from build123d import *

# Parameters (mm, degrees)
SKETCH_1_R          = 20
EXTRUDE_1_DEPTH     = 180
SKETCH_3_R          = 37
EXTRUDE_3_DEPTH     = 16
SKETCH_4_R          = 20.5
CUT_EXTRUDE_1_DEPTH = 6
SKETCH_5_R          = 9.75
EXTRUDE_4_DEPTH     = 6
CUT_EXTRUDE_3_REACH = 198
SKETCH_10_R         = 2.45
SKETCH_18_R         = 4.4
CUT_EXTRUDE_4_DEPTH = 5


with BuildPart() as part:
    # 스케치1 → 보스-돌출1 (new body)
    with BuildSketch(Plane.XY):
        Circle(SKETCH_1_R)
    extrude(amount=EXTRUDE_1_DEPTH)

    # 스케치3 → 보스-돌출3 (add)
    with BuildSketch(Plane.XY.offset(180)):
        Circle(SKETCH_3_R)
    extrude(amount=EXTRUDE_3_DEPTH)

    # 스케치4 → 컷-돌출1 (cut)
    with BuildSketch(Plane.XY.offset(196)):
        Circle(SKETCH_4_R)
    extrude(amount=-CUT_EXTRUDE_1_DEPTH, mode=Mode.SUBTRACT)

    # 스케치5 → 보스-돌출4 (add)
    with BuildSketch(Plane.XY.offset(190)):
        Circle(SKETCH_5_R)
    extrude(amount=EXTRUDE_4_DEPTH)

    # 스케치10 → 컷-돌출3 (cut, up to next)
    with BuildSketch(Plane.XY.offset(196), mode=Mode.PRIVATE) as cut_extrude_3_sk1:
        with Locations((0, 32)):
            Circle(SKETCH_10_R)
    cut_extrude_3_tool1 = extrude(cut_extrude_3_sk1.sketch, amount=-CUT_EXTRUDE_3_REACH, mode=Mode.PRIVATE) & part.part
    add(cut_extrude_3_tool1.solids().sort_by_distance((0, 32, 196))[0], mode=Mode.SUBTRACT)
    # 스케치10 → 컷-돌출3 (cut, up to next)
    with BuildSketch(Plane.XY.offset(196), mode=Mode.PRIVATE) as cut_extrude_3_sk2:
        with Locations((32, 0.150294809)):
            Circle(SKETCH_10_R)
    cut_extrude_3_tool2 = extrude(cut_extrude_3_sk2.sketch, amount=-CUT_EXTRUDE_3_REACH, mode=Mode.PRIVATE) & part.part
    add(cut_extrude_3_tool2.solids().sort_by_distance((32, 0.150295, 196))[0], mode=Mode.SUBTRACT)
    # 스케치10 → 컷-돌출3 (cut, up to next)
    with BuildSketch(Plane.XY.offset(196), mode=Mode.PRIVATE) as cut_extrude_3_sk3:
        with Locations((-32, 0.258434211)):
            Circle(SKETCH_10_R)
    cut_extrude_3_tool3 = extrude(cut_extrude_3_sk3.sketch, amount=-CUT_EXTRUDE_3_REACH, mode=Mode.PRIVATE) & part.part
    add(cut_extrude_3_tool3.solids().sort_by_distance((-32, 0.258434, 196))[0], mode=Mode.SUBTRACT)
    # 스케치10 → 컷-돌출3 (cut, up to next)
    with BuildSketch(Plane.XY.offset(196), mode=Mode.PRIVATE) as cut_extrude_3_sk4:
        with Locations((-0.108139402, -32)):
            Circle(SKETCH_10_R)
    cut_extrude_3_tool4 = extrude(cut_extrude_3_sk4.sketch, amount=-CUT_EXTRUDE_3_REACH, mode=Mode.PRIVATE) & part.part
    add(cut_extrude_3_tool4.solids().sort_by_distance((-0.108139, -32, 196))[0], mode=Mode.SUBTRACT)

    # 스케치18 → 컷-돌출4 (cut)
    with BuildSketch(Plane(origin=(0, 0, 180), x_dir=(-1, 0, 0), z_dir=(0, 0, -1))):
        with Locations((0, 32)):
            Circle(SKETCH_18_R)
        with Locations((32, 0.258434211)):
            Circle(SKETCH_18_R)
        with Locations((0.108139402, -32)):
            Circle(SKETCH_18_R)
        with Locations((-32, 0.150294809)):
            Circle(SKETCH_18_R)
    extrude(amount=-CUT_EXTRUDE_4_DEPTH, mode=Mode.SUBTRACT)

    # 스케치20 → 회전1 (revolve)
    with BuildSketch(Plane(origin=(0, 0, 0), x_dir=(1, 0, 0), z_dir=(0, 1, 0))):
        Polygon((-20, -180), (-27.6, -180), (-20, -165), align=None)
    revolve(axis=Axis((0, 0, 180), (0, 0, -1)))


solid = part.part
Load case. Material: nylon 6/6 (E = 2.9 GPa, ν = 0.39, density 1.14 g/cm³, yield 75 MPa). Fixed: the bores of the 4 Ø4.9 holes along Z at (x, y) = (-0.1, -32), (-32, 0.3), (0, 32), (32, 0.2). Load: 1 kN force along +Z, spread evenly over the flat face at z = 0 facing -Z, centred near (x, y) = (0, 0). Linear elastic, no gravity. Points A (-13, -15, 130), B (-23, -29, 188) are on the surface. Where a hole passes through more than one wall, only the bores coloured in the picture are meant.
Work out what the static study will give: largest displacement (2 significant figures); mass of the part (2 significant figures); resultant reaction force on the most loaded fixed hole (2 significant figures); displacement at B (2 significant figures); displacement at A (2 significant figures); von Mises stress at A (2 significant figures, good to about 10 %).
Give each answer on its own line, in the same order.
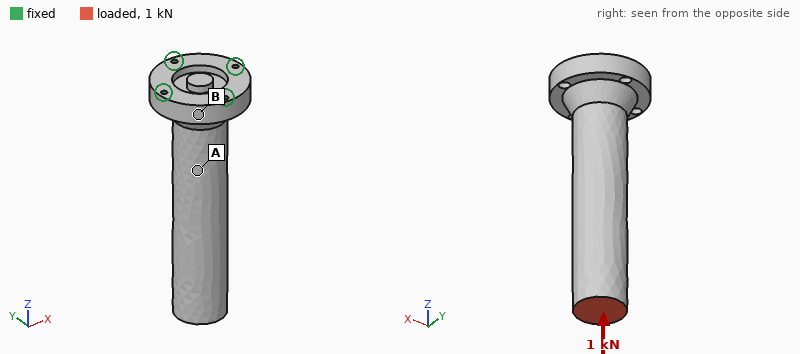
61 µm
340 g
280 N
9.9 µm
25 µm
0.80 MPa
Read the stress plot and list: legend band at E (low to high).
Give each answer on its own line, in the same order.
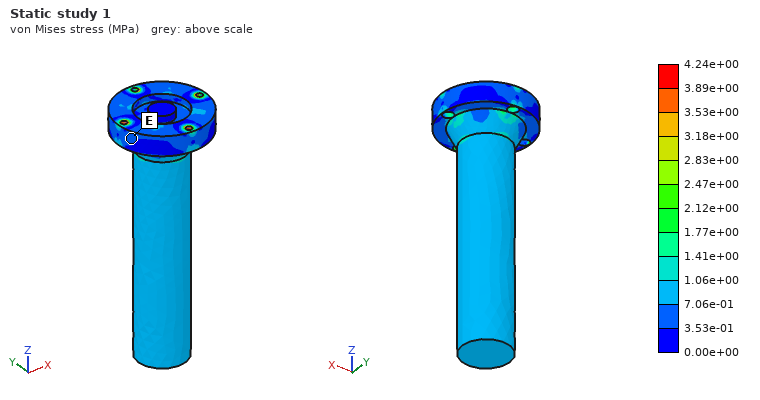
3.53e-01 to 7.06e-01 MPa
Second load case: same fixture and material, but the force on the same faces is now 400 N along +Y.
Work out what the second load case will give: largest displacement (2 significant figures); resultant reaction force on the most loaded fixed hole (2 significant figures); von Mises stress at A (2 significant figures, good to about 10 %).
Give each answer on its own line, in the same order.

2.4 mm
1.3 kN
6.5 MPa
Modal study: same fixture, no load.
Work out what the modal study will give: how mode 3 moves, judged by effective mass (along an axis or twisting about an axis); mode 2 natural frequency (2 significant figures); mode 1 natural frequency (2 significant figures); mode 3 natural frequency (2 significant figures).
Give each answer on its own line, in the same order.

twisting about Z
250 Hz
250 Hz
1300 Hz
